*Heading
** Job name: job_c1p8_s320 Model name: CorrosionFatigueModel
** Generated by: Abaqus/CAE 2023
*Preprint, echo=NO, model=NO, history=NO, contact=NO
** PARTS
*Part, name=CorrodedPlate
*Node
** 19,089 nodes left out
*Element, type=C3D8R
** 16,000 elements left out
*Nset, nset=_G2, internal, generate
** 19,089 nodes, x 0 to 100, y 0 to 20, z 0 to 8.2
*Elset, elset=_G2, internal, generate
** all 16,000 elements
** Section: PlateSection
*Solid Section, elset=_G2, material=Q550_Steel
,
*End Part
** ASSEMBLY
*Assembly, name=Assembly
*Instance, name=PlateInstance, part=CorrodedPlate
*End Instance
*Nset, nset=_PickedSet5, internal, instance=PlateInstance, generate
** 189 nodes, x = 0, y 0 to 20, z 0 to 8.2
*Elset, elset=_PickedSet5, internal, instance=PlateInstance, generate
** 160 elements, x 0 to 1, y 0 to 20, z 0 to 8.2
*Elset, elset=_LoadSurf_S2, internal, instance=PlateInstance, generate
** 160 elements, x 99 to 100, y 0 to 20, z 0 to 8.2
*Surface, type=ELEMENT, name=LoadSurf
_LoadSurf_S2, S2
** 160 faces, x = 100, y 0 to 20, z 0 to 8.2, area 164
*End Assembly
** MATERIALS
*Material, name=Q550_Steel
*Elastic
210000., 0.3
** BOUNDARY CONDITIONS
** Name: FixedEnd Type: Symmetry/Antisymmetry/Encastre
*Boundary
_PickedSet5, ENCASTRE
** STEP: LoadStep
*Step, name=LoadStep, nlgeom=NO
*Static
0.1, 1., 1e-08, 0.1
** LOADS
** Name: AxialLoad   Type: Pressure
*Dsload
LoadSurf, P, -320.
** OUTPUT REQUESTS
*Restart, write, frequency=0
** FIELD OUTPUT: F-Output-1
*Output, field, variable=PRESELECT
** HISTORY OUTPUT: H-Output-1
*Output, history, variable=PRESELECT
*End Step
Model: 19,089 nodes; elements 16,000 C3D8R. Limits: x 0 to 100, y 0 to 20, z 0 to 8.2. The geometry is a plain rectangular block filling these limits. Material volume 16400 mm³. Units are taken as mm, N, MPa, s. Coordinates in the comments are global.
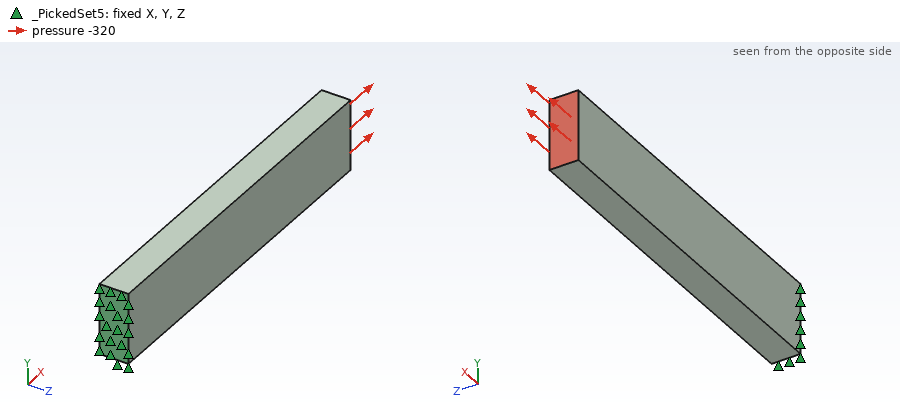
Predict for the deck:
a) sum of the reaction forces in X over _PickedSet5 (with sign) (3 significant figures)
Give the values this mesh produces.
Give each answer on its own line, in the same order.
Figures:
-52500 N
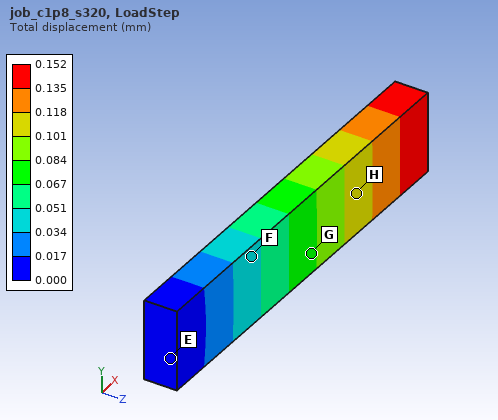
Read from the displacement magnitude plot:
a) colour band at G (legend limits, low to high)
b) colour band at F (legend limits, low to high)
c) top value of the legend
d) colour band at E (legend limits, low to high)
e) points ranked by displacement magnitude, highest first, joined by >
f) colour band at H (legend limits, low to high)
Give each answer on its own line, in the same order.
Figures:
0.067 to 0.084 mm
0.034 to 0.051 mm
0.152 mm
0.000 to 0.017 mm
H > G > F > E
0.101 to 0.118 mm
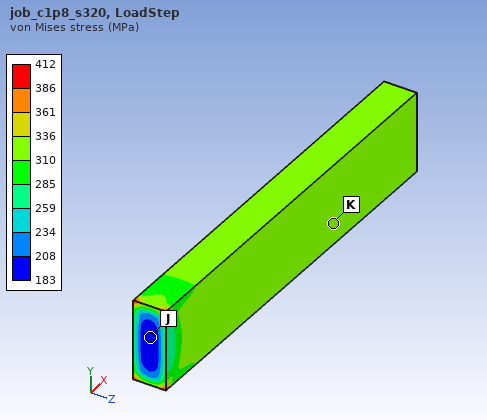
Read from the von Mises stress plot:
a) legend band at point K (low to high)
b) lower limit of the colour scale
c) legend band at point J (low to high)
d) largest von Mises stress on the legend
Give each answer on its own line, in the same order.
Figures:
310 to 336 MPa
183 MPa
183 to 208 MPa
412 MPa
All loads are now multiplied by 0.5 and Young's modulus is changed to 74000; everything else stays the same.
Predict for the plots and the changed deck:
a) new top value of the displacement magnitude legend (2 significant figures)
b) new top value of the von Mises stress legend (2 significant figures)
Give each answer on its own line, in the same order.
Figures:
0.22 mm
210 MPa
